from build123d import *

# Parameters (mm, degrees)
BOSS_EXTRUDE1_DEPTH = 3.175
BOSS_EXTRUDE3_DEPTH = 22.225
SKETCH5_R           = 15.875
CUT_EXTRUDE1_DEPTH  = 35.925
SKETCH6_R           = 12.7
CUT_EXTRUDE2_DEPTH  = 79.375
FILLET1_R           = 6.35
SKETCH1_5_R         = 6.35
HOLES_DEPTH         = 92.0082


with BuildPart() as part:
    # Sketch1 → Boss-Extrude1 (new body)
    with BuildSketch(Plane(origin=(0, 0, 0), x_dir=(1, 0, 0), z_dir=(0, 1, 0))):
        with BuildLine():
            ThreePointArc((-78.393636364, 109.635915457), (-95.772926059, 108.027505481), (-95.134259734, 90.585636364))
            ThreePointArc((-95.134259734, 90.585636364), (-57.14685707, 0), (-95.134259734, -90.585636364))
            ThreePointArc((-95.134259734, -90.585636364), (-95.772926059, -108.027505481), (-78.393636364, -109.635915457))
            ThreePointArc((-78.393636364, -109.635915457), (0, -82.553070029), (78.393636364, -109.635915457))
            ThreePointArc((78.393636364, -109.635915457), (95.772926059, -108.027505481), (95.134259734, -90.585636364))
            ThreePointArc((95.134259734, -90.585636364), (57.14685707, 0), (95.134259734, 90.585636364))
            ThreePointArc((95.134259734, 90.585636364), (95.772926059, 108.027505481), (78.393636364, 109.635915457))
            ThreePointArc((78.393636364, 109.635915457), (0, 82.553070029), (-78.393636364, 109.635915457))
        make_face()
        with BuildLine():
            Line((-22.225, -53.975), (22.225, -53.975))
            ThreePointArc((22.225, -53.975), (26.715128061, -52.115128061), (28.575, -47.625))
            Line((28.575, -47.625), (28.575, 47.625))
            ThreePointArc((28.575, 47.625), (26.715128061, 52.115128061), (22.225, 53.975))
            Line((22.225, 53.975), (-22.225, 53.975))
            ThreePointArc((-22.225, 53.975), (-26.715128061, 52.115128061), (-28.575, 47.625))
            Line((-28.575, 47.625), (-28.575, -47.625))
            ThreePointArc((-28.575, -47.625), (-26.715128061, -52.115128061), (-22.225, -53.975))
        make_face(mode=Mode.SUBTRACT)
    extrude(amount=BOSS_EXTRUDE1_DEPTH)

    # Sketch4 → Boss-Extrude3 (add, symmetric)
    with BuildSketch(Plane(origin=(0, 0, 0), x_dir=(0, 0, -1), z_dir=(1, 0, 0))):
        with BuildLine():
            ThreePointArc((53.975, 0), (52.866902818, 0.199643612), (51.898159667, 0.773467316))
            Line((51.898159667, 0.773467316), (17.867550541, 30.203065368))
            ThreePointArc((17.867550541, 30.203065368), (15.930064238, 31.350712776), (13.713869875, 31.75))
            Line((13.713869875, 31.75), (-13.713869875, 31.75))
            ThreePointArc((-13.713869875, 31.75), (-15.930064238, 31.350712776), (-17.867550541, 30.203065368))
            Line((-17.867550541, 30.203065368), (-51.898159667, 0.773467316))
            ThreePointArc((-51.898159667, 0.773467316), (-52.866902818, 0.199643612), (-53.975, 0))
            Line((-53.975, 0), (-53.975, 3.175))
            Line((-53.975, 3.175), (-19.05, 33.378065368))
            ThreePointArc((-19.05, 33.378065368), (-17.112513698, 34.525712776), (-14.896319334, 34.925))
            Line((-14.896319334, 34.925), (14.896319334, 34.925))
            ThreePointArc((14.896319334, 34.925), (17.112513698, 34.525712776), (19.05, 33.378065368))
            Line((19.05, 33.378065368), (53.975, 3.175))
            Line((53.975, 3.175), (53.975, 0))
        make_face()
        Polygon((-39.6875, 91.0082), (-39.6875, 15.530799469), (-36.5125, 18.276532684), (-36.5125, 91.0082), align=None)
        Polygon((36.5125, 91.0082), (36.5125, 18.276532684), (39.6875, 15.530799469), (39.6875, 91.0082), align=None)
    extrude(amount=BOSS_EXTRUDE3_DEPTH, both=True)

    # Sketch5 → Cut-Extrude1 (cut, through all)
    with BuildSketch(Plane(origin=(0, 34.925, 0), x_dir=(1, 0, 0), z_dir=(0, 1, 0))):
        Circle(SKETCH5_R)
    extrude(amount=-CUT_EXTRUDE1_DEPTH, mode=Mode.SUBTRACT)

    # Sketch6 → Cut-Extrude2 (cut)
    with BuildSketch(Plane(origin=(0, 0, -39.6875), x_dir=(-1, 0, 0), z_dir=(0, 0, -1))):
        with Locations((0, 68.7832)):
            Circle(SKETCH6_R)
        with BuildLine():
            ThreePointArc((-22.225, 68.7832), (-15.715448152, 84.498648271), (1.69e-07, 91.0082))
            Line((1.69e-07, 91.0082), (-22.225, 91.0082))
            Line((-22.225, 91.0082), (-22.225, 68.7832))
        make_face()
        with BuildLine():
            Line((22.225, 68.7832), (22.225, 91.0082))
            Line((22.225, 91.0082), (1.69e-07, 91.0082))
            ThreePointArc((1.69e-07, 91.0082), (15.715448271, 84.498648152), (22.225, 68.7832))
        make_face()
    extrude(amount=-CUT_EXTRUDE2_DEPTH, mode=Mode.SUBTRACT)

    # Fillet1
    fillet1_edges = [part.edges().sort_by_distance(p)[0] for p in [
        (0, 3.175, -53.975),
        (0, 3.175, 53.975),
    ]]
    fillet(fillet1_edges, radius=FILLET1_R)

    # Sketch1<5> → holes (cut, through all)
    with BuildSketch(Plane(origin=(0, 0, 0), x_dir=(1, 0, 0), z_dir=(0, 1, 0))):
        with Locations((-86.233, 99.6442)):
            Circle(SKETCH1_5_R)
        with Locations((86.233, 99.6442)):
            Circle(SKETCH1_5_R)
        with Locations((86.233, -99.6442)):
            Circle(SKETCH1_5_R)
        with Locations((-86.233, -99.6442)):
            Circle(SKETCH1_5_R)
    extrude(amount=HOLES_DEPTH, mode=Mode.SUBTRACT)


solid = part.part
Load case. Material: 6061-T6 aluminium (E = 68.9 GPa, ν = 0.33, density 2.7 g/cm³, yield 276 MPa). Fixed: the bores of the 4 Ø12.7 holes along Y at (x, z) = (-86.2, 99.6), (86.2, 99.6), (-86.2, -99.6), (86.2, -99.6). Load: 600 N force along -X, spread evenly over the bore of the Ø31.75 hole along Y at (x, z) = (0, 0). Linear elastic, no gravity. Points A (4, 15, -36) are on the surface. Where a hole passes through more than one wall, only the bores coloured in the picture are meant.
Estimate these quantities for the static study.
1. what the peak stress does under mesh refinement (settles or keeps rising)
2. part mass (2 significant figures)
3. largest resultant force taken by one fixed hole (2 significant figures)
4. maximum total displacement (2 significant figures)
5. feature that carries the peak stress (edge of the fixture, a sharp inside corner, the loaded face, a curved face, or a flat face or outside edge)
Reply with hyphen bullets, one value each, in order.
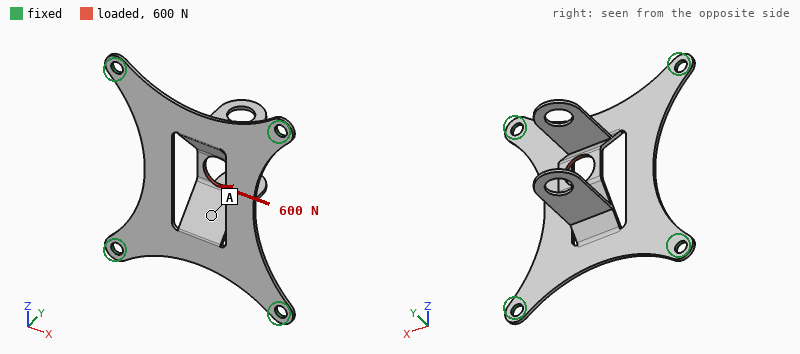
- keeps rising
- 260 g
- 190 N
- 1.2 mm
- a sharp inside corner
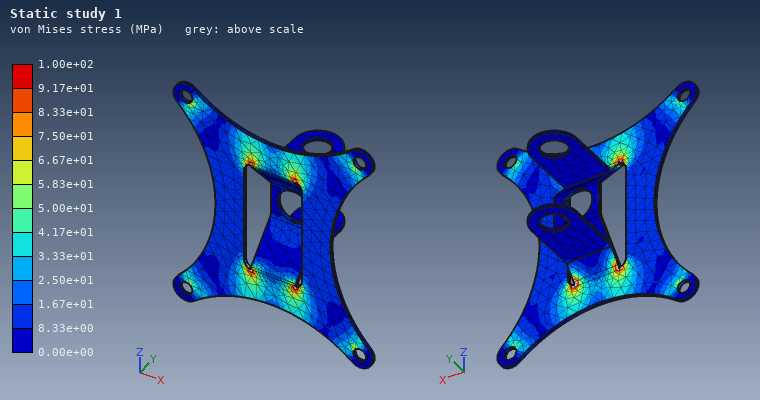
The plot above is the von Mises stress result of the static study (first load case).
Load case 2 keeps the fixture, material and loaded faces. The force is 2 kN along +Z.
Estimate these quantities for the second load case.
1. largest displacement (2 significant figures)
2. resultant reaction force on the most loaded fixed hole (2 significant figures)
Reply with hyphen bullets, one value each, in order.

- 2.2 mm
- 720 N
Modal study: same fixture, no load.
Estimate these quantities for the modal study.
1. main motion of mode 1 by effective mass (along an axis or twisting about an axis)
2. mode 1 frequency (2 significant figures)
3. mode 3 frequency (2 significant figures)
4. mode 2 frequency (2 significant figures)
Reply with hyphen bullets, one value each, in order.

- along Y
- 260 Hz
- 410 Hz
- 390 Hz
